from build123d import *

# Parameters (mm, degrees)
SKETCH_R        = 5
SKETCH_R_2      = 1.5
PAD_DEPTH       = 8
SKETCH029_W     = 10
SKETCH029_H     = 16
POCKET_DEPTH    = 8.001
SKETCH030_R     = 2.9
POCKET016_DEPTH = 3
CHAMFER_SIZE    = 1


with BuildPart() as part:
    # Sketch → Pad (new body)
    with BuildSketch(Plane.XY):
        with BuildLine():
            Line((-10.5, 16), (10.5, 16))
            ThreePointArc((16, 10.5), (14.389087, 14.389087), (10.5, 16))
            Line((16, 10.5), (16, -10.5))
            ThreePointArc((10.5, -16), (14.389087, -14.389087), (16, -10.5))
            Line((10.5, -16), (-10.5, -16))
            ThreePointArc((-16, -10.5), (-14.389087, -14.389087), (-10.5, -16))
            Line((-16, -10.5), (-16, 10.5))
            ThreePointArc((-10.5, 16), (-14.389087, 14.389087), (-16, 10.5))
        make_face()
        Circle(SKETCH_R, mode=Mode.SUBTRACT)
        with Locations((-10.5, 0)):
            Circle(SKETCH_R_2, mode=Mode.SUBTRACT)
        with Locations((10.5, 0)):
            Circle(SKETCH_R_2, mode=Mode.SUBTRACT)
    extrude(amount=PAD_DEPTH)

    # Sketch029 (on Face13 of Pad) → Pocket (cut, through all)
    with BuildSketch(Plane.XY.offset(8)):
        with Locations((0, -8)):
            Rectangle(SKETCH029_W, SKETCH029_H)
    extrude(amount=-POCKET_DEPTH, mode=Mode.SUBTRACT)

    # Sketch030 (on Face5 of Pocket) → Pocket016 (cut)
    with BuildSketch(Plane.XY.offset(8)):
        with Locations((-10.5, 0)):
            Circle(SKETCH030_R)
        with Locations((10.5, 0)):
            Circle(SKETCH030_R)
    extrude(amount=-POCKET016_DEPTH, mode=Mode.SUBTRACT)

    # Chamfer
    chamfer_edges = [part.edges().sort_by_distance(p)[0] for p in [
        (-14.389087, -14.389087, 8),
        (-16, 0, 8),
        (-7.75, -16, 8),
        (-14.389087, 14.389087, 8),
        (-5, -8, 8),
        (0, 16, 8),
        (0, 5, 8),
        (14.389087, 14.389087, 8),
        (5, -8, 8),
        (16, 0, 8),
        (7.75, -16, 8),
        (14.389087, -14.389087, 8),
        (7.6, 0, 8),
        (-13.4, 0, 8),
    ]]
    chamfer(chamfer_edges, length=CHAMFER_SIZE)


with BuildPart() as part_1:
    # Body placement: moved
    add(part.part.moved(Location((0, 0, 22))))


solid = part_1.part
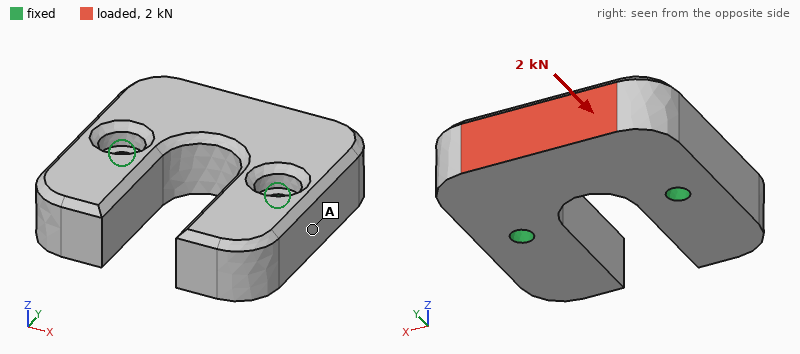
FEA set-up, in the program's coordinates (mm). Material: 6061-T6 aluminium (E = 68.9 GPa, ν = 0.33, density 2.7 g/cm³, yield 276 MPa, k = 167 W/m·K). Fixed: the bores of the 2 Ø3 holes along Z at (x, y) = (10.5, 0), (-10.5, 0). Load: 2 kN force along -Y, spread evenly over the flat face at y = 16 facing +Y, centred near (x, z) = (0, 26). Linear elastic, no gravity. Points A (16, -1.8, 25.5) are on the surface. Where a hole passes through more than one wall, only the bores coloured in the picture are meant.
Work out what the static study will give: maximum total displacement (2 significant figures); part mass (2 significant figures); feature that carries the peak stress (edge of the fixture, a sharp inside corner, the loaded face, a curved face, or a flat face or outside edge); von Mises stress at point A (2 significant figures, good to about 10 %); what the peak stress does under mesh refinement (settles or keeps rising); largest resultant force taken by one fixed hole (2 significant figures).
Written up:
5.9 µm
16 g
edge of the fixture
7.9 MPa
keeps rising
1.1 kN
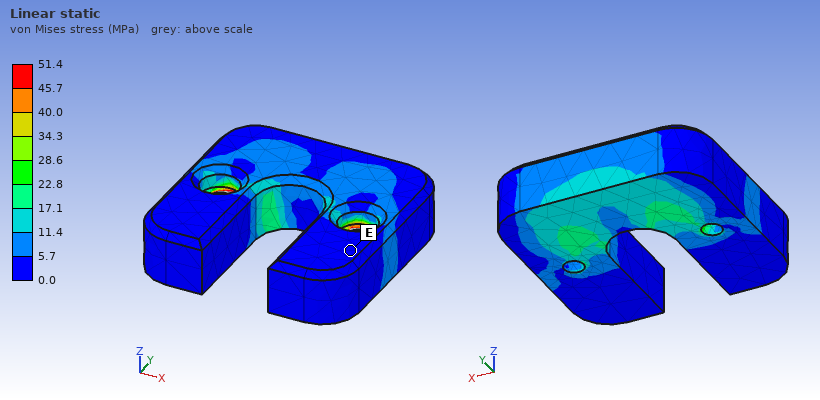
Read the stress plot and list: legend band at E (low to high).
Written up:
0.0 to 5.7 MPa
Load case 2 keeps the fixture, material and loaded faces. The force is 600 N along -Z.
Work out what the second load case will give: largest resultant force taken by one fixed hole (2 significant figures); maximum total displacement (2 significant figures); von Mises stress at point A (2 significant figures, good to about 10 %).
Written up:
300 N
32 µm
15 MPa
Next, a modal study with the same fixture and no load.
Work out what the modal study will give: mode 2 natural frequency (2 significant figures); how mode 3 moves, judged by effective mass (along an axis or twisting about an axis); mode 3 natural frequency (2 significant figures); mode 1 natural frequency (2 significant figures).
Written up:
16 kHz
along Z
19 kHz
12 kHz
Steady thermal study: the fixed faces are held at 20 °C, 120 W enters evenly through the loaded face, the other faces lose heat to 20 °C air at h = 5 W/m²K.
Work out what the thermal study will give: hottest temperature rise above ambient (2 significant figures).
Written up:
74 K
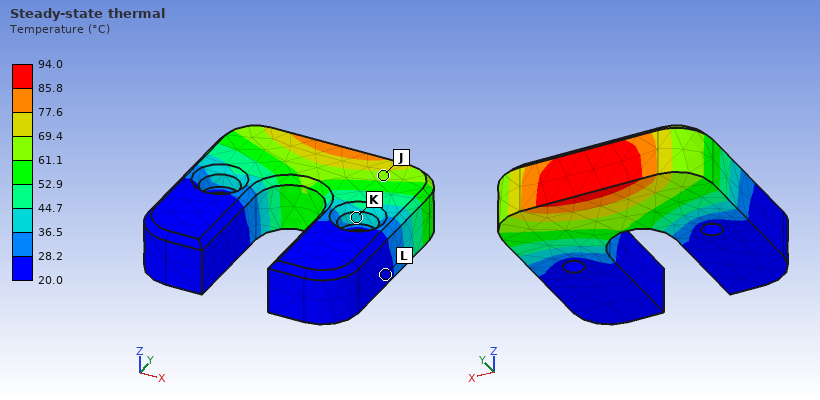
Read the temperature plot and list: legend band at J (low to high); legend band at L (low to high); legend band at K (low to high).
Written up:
61.1 to 69.4 °C
20.0 to 28.2 °C
36.5 to 44.7 °C
